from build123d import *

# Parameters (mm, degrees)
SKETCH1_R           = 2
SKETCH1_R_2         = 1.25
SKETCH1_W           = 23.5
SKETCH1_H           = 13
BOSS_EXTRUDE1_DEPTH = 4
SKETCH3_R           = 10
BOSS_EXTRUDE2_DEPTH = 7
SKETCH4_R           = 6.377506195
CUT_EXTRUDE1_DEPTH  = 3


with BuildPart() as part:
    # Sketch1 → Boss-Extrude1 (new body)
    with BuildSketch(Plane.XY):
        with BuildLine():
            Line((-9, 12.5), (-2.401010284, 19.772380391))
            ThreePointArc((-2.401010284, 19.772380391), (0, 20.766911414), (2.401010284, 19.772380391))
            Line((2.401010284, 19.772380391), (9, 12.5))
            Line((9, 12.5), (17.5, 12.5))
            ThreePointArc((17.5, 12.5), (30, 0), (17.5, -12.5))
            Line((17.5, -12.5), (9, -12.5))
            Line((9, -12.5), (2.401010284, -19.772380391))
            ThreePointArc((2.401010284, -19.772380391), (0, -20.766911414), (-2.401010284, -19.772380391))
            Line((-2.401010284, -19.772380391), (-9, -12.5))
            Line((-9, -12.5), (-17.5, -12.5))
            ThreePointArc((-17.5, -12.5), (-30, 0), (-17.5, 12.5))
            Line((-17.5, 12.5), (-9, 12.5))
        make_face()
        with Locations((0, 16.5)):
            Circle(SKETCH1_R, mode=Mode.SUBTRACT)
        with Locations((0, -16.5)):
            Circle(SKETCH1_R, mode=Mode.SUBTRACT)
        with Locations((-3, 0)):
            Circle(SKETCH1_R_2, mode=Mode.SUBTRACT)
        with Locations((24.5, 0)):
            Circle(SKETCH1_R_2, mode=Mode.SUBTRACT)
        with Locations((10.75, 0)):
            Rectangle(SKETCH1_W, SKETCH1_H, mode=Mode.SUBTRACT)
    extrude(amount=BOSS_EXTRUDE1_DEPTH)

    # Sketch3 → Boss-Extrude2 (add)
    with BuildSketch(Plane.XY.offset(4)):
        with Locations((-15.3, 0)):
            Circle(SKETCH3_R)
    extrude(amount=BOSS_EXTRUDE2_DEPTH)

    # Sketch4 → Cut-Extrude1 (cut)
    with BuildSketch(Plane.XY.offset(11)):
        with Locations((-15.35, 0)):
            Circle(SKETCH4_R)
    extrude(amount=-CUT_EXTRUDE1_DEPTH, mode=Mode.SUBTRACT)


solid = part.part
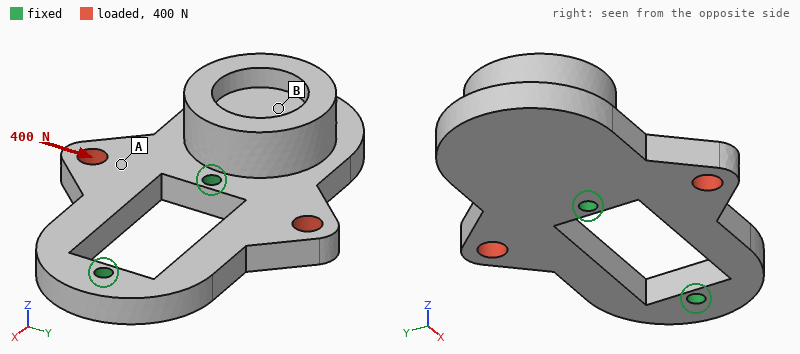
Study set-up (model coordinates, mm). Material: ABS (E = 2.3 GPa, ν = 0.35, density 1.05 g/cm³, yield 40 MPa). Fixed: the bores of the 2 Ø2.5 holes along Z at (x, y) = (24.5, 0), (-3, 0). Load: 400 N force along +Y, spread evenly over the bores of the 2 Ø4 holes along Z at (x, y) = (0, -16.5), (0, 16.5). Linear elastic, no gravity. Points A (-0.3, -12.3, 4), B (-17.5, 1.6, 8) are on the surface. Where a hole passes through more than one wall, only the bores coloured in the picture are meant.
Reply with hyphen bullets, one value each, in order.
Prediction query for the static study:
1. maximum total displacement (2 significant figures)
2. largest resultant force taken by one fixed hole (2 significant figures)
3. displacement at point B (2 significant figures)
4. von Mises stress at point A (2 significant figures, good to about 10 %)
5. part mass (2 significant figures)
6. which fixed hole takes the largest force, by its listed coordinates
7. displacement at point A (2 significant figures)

- 92 µm
- 360 N
- 17 µm
- 6.0 MPa
- 6.9 g
- (-3, 0)
- 57 µm
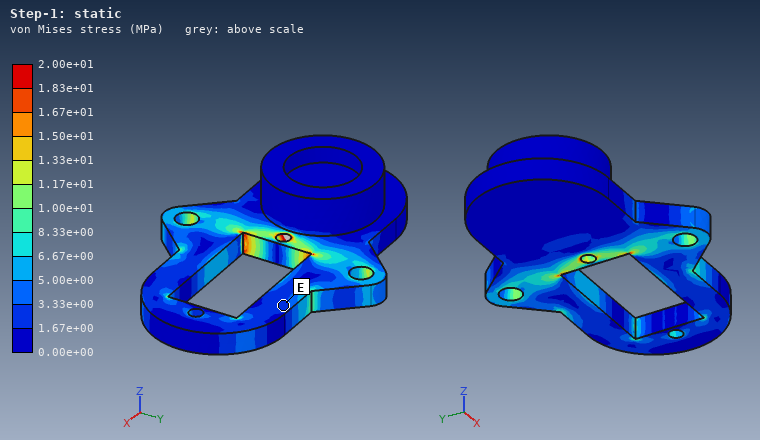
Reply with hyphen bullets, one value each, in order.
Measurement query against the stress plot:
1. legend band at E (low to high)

- 1.67e+00 to 3.33e+00 MPa
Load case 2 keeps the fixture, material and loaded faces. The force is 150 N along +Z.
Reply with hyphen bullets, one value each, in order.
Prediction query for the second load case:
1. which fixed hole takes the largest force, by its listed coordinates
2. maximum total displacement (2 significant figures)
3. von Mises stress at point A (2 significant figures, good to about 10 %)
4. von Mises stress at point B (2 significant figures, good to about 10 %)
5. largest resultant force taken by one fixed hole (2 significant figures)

- (-3, 0)
- 0.67 mm
- 11 MPa
- 2.4 MPa
- 130 N
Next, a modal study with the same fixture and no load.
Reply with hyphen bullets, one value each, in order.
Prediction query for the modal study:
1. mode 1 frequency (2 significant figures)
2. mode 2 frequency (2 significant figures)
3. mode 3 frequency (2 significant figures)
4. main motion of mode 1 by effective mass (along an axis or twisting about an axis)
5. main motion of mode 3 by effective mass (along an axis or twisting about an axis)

- 1100 Hz
- 1800 Hz
- 2200 Hz
- along Z
- along Y
